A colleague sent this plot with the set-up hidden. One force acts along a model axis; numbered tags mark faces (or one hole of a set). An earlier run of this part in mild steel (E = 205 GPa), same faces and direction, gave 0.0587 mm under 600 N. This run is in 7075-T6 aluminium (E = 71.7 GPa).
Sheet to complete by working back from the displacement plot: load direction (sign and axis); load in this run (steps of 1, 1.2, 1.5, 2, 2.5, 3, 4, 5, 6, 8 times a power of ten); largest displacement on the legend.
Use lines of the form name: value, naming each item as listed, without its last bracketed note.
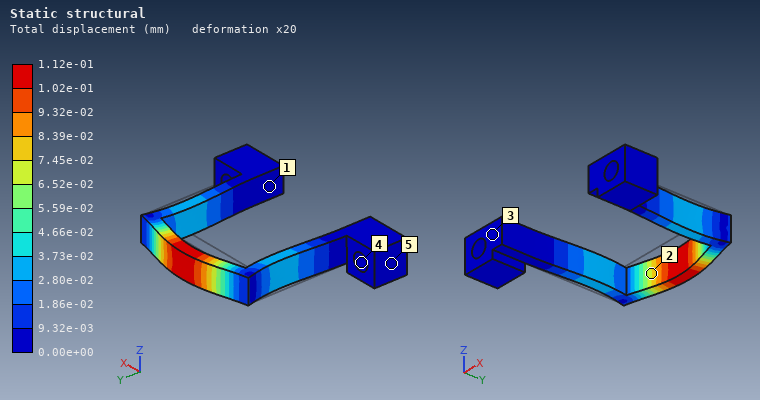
load direction: +Y
load in this run: 400 N
largest displacement on the legend: 1.12e-01 mm
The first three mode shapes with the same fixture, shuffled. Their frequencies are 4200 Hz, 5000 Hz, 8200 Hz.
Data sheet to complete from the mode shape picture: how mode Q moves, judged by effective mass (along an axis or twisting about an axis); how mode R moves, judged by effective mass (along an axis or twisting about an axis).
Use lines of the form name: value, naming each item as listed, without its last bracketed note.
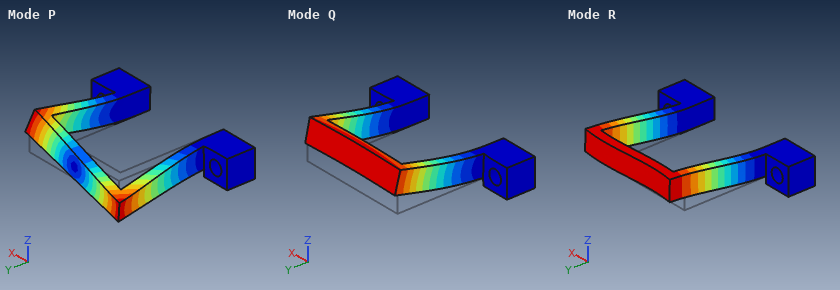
how mode Q moves, judged by effective mass: along Z
how mode R moves, judged by effective mass: along X
